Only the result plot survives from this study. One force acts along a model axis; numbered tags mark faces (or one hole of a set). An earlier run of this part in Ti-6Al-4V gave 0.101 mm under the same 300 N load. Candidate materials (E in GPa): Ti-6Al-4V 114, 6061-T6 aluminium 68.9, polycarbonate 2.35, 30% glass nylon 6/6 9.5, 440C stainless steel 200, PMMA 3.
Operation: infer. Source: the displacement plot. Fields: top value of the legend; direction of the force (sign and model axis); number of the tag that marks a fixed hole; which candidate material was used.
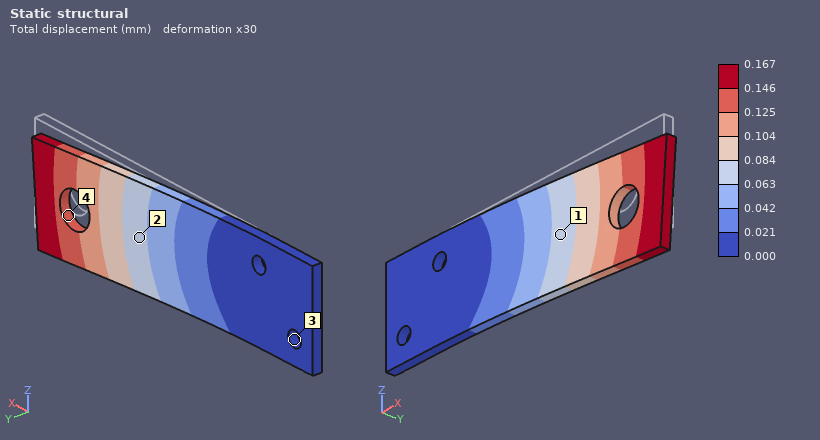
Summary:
0.167 mm
-Z
3
6061-T6 aluminium
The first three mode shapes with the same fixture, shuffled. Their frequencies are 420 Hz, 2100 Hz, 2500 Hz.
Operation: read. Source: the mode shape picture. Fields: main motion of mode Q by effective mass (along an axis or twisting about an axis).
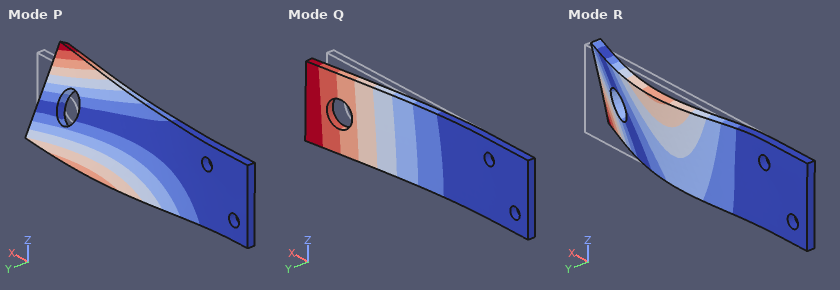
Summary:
along Y
